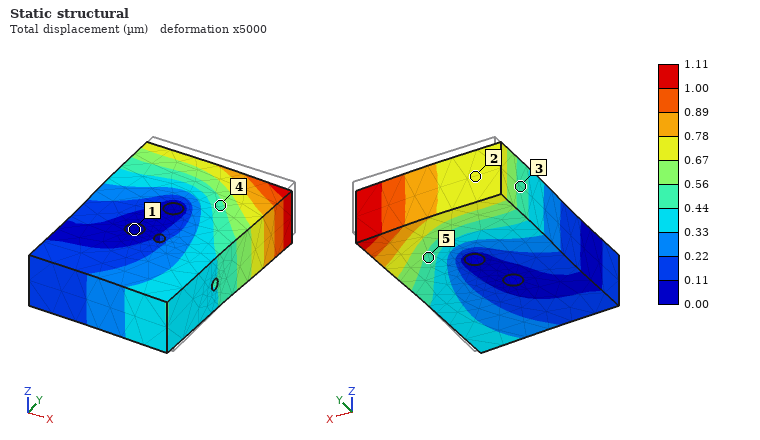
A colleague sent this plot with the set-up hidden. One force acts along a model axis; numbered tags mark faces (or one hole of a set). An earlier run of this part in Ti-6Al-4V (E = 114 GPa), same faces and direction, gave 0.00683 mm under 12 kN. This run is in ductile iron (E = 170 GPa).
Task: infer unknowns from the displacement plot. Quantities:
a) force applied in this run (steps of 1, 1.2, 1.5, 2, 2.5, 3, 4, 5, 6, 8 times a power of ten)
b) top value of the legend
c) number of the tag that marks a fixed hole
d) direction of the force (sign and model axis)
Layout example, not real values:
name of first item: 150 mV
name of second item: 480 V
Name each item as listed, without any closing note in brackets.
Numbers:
force applied in this run: 3 kN
top value of the legend: 1.11 µm
number of the tag that marks a fixed hole: 1
direction of the force: -Y
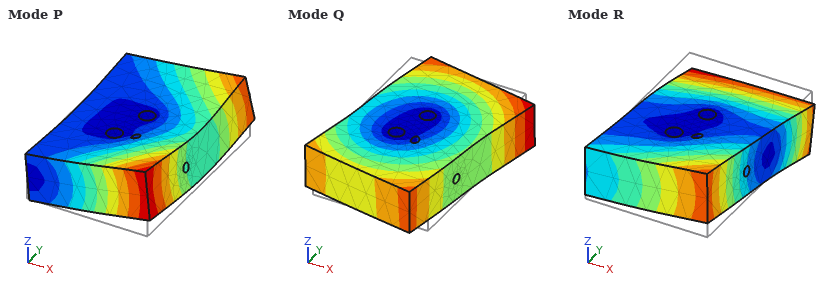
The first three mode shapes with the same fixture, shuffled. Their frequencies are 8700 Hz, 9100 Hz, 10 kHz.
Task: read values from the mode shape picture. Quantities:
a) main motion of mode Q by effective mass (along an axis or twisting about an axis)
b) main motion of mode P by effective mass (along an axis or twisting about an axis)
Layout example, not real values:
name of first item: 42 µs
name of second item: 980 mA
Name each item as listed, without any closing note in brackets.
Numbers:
main motion of mode Q by effective mass: twisting about Z
main motion of mode P by effective mass: along Z
